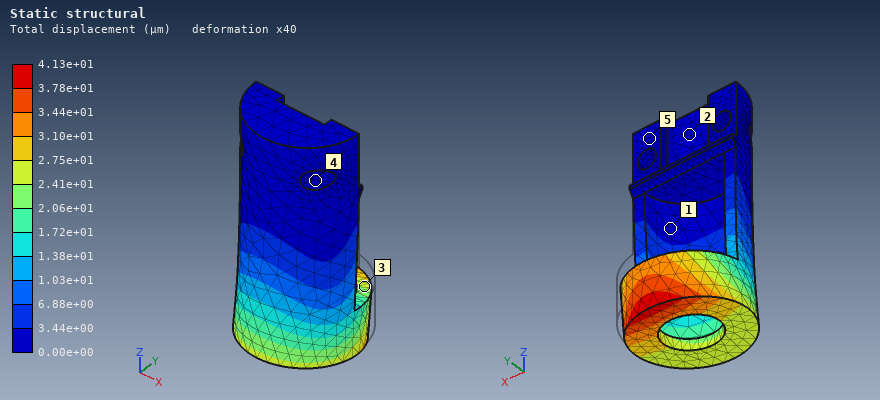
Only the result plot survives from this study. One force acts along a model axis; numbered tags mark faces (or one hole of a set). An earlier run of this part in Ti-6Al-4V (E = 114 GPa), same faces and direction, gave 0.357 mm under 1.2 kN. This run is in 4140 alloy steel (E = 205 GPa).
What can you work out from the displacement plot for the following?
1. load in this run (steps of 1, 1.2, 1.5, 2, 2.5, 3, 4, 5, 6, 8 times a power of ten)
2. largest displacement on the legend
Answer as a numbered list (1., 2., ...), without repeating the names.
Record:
1. 250 N
2. 4.13e+01 µm
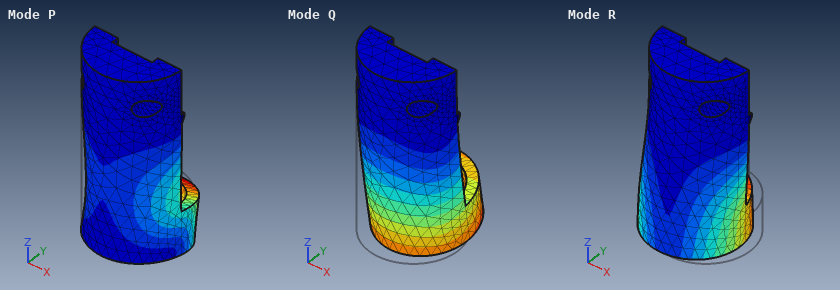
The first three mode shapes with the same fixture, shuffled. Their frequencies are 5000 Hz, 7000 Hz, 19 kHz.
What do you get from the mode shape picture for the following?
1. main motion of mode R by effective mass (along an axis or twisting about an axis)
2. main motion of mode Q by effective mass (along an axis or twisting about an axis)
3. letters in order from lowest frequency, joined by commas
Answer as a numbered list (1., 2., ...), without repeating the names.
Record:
1. along X
2. along Y
3. R, Q, P
